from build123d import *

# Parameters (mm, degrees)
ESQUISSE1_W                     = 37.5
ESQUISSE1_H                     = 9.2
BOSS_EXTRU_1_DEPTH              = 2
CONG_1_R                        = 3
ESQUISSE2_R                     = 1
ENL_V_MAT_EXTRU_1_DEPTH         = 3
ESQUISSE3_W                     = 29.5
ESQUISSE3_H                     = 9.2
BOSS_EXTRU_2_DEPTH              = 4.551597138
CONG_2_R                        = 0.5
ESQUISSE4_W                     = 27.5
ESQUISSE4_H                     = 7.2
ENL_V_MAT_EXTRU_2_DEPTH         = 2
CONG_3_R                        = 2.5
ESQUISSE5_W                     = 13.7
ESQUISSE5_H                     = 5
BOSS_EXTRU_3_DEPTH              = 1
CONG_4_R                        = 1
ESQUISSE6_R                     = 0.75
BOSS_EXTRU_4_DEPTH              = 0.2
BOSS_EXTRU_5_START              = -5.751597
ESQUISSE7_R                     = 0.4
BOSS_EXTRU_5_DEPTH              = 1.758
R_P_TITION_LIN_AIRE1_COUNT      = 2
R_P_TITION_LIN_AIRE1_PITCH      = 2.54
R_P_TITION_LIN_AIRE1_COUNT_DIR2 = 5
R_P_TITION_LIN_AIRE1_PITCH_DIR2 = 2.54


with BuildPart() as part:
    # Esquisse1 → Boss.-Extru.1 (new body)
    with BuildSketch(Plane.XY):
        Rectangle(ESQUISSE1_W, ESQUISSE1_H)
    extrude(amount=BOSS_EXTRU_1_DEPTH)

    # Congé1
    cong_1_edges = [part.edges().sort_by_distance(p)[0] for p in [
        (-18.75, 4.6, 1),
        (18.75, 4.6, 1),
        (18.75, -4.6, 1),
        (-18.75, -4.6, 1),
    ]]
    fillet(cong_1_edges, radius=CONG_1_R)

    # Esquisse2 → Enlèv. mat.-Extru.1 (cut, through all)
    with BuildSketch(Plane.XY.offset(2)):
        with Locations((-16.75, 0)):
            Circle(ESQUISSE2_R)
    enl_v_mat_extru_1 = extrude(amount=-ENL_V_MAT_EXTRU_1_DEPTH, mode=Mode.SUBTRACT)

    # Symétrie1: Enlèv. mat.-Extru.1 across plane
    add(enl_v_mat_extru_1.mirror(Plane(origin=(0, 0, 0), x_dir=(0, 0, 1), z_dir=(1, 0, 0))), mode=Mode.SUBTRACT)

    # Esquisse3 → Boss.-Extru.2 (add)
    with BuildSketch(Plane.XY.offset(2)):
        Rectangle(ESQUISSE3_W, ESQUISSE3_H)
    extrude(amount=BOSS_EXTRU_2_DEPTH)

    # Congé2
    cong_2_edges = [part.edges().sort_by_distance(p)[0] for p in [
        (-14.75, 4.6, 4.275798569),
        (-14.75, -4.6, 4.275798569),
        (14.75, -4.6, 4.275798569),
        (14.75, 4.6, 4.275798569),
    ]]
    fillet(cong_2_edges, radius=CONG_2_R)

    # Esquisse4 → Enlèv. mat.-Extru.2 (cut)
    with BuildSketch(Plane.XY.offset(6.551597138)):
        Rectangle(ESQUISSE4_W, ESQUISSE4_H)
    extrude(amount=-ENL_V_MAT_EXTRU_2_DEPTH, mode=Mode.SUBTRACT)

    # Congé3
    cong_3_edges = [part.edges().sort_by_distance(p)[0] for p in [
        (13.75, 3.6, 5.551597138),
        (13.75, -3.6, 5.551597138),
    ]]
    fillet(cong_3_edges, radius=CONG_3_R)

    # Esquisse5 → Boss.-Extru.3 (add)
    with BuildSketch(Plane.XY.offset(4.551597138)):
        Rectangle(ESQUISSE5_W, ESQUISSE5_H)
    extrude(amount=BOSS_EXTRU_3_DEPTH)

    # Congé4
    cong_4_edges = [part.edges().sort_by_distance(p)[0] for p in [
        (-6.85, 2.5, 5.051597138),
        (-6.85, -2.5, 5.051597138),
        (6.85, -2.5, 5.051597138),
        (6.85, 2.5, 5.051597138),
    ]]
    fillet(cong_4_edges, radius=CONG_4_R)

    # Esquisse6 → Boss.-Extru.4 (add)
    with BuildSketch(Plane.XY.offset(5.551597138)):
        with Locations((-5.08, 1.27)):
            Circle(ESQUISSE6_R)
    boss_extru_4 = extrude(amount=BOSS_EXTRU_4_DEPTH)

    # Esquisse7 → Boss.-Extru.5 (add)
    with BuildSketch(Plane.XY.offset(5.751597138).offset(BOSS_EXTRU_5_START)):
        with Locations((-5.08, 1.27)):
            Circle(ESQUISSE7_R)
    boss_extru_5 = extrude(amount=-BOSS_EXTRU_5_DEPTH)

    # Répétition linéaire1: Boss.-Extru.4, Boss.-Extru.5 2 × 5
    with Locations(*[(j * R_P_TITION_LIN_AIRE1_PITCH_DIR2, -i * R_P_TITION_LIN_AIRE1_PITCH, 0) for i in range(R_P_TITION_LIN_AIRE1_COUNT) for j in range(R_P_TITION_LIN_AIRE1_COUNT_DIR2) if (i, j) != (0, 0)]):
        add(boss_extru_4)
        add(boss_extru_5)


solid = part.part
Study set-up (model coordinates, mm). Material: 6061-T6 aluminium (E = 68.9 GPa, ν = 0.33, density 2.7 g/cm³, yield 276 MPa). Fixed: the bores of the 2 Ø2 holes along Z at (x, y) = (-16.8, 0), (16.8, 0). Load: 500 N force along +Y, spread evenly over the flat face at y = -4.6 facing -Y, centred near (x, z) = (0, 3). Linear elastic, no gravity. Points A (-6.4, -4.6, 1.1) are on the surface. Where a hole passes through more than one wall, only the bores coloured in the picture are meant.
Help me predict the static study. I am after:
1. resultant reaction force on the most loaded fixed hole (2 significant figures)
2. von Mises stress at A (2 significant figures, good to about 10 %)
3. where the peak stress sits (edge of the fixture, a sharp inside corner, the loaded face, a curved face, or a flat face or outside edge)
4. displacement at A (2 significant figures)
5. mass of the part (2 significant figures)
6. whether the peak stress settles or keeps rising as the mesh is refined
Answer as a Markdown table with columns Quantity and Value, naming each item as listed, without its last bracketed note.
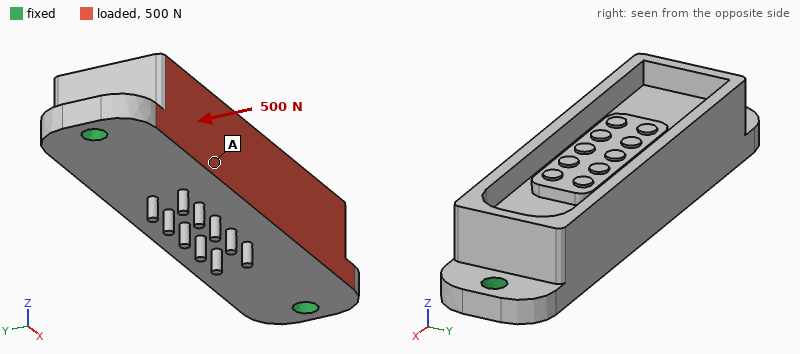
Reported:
| Quantity | Value |
|---|---|
| resultant reaction force on the most loaded fixed hole | 250 N |
| von Mises stress at A | 21 MPa |
| where the peak stress sits | edge of the fixture |
| displacement at A | 15 µm |
| mass of the part | 4.3 g |
| whether the peak stress settles or keeps rising as the mesh is refined | keeps rising |
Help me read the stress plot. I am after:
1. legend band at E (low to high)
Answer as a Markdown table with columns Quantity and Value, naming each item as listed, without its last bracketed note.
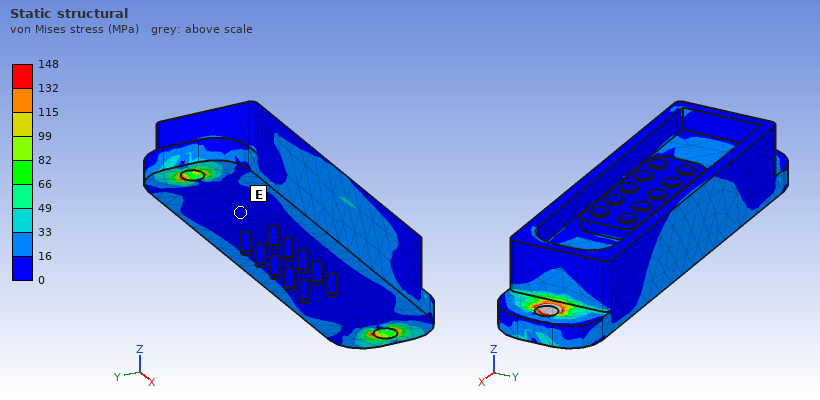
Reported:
| Quantity | Value |
|---|---|
| legend band at E | 0 to 16 MPa |
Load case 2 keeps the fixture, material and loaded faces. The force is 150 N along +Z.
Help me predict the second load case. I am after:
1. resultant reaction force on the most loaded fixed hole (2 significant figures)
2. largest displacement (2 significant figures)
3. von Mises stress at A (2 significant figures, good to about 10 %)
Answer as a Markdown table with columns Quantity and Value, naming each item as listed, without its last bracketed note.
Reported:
| Quantity | Value |
|---|---|
| resultant reaction force on the most loaded fixed hole | 110 N |
| largest displacement | 17 µm |
| von Mises stress at A | 5.0 MPa |
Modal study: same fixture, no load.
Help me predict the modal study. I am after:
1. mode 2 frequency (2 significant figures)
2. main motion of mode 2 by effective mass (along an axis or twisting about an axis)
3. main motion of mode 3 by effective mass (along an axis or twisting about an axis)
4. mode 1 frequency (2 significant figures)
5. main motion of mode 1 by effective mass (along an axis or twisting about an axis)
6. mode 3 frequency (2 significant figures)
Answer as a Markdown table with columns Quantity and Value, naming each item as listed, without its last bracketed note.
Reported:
| Quantity | Value |
|---|---|
| mode 2 frequency | 15 kHz |
| main motion of mode 2 by effective mass | along Z |
| main motion of mode 3 by effective mass | along Y |
| mode 1 frequency | 13 kHz |
| main motion of mode 1 by effective mass | along Y |
| mode 3 frequency | 22 kHz |
